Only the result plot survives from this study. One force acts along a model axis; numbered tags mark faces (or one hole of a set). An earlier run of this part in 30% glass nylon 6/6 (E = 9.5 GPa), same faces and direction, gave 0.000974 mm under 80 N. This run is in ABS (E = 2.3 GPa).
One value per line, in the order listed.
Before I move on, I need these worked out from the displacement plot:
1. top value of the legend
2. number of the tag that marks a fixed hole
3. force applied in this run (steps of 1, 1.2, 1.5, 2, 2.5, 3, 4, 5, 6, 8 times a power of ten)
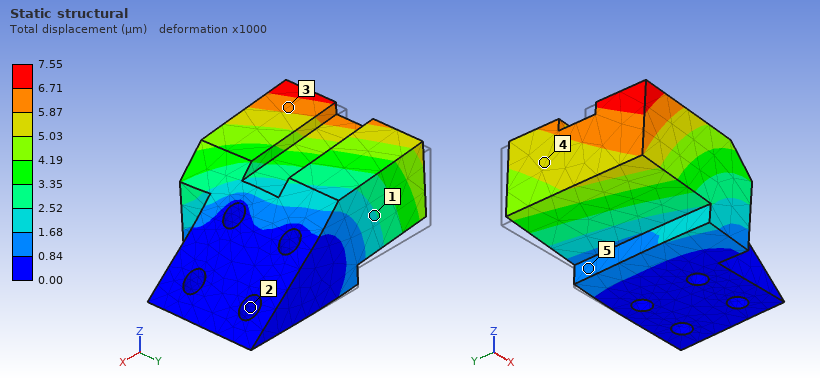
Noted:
7.55 µm
2
150 N
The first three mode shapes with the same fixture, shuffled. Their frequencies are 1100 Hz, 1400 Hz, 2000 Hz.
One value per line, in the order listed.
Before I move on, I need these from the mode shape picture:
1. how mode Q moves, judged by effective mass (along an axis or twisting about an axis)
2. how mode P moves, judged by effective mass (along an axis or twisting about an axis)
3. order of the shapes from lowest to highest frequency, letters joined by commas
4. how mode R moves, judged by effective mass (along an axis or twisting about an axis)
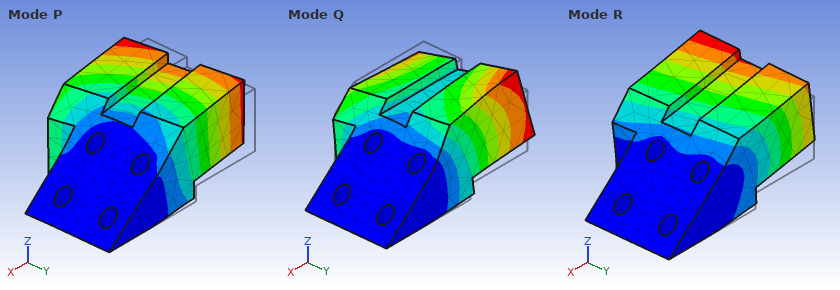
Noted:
twisting about X
along Y
R, P, Q
along Z
